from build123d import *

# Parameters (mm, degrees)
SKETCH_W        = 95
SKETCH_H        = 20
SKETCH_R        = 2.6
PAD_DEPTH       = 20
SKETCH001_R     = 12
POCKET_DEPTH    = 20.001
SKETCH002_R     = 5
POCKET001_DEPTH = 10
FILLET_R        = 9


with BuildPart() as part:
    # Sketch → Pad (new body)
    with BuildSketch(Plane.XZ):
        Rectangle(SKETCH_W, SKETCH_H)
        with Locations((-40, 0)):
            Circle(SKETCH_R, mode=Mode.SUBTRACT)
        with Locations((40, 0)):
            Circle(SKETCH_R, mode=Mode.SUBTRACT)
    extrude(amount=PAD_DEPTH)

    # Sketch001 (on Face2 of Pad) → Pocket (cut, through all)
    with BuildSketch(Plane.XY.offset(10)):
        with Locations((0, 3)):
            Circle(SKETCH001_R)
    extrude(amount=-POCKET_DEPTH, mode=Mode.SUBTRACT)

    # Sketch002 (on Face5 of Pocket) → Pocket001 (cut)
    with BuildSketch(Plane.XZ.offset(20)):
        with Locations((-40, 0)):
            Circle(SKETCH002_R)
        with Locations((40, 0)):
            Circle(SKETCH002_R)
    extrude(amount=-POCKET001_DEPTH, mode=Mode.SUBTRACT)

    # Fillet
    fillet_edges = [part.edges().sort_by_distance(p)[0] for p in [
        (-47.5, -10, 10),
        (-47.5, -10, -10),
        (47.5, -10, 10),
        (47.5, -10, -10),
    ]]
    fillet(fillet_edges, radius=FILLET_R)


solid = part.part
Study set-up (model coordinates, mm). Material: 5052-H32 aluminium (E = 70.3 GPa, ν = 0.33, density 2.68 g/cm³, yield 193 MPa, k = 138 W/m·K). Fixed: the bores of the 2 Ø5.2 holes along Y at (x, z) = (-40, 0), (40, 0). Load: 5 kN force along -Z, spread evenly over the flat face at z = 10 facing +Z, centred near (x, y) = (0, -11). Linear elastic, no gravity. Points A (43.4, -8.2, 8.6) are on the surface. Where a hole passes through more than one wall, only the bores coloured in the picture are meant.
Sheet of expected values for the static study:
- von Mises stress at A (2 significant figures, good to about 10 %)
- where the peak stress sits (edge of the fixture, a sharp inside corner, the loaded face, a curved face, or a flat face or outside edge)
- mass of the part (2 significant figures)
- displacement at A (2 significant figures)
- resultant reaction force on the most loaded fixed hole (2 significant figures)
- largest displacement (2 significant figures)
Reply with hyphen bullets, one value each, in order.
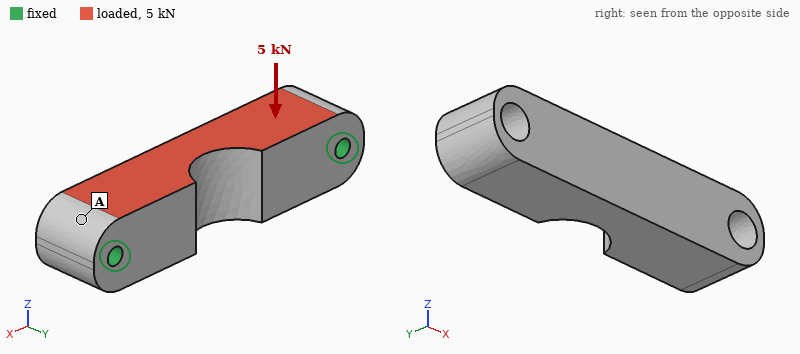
- 18 MPa
- edge of the fixture
- 84 g
- 7.4 µm
- 2.5 kN
- 43 µm
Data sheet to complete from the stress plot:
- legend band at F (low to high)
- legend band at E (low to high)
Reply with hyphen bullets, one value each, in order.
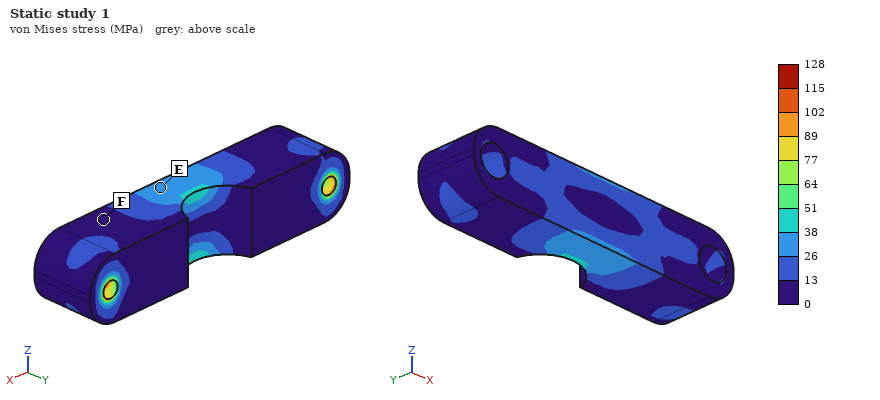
- 0 to 13 MPa
- 26 to 38 MPa
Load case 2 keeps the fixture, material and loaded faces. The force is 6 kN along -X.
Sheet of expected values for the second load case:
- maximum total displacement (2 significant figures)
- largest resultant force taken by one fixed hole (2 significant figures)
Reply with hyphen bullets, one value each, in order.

- 7.0 µm
- 3.1 kN
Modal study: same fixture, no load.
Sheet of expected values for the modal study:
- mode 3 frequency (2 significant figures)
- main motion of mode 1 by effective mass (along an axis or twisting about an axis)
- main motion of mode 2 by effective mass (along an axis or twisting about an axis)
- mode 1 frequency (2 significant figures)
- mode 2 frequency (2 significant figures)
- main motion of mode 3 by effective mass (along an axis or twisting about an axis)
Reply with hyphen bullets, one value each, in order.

- 15 kHz
- along Z
- along Y
- 7700 Hz
- 9400 Hz
- twisting about X
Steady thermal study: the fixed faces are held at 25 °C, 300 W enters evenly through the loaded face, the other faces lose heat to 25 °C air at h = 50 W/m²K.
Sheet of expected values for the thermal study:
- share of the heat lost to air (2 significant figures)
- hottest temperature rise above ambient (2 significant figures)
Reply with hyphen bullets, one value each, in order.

- 4.6 %
- 79 K
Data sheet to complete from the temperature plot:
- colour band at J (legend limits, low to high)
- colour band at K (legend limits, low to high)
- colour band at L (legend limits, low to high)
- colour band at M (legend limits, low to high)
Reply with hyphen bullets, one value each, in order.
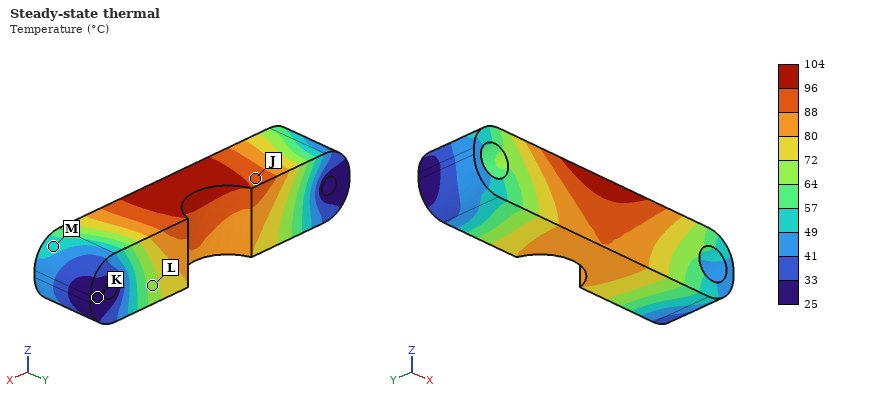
- 88 to 96 °C
- 25 to 33 °C
- 64 to 72 °C
- 49 to 57 °C
